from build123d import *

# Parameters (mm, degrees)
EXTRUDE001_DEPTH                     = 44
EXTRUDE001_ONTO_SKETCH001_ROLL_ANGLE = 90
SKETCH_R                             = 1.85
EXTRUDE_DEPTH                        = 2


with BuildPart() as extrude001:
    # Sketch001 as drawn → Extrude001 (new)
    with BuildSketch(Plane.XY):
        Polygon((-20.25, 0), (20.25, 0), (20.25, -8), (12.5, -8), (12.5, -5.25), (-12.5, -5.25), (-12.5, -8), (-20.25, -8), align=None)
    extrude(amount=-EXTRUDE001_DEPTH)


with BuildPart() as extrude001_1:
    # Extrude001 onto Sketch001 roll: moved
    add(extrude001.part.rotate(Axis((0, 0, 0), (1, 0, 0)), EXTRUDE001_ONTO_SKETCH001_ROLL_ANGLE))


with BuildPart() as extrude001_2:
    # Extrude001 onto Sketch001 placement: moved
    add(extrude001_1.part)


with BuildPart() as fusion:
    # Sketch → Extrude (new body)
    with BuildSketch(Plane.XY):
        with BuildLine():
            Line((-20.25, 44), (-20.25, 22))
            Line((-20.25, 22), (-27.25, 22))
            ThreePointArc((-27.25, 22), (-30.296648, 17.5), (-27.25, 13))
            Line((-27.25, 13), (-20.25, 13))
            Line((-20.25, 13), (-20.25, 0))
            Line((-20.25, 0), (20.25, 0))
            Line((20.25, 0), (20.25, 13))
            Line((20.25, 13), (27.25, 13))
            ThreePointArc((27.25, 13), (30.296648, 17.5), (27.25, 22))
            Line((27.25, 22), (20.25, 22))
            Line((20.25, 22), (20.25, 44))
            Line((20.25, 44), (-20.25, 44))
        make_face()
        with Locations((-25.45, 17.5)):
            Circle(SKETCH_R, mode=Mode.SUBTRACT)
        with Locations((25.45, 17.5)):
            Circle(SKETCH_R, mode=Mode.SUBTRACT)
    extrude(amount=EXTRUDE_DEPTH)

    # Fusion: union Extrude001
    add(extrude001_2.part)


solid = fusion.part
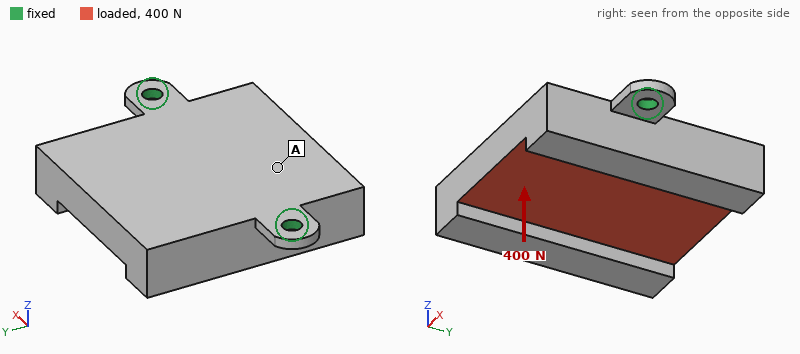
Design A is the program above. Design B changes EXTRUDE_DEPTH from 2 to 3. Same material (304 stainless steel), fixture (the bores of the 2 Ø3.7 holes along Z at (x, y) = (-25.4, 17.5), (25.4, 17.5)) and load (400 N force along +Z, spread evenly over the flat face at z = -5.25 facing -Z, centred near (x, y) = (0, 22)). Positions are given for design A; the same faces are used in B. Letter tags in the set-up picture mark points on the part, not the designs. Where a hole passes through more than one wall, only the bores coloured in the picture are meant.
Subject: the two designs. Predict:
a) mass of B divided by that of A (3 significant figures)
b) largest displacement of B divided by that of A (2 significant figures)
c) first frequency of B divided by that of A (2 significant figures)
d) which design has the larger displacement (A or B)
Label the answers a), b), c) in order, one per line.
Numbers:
a) 1.13
b) 0.44
c) 1.5
d) A
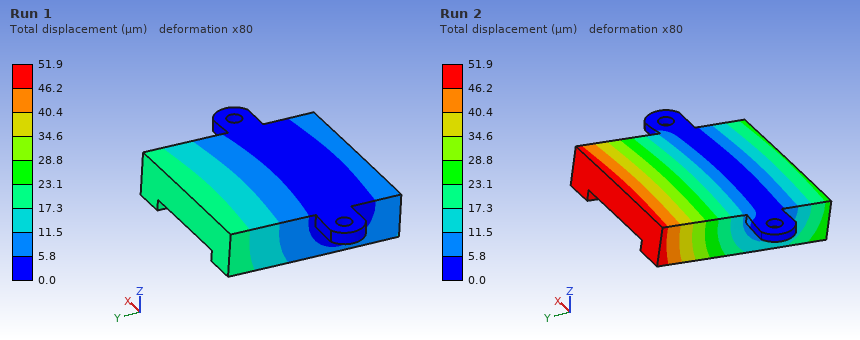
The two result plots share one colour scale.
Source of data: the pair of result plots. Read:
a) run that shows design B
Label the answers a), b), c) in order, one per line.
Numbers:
a) Run 1
